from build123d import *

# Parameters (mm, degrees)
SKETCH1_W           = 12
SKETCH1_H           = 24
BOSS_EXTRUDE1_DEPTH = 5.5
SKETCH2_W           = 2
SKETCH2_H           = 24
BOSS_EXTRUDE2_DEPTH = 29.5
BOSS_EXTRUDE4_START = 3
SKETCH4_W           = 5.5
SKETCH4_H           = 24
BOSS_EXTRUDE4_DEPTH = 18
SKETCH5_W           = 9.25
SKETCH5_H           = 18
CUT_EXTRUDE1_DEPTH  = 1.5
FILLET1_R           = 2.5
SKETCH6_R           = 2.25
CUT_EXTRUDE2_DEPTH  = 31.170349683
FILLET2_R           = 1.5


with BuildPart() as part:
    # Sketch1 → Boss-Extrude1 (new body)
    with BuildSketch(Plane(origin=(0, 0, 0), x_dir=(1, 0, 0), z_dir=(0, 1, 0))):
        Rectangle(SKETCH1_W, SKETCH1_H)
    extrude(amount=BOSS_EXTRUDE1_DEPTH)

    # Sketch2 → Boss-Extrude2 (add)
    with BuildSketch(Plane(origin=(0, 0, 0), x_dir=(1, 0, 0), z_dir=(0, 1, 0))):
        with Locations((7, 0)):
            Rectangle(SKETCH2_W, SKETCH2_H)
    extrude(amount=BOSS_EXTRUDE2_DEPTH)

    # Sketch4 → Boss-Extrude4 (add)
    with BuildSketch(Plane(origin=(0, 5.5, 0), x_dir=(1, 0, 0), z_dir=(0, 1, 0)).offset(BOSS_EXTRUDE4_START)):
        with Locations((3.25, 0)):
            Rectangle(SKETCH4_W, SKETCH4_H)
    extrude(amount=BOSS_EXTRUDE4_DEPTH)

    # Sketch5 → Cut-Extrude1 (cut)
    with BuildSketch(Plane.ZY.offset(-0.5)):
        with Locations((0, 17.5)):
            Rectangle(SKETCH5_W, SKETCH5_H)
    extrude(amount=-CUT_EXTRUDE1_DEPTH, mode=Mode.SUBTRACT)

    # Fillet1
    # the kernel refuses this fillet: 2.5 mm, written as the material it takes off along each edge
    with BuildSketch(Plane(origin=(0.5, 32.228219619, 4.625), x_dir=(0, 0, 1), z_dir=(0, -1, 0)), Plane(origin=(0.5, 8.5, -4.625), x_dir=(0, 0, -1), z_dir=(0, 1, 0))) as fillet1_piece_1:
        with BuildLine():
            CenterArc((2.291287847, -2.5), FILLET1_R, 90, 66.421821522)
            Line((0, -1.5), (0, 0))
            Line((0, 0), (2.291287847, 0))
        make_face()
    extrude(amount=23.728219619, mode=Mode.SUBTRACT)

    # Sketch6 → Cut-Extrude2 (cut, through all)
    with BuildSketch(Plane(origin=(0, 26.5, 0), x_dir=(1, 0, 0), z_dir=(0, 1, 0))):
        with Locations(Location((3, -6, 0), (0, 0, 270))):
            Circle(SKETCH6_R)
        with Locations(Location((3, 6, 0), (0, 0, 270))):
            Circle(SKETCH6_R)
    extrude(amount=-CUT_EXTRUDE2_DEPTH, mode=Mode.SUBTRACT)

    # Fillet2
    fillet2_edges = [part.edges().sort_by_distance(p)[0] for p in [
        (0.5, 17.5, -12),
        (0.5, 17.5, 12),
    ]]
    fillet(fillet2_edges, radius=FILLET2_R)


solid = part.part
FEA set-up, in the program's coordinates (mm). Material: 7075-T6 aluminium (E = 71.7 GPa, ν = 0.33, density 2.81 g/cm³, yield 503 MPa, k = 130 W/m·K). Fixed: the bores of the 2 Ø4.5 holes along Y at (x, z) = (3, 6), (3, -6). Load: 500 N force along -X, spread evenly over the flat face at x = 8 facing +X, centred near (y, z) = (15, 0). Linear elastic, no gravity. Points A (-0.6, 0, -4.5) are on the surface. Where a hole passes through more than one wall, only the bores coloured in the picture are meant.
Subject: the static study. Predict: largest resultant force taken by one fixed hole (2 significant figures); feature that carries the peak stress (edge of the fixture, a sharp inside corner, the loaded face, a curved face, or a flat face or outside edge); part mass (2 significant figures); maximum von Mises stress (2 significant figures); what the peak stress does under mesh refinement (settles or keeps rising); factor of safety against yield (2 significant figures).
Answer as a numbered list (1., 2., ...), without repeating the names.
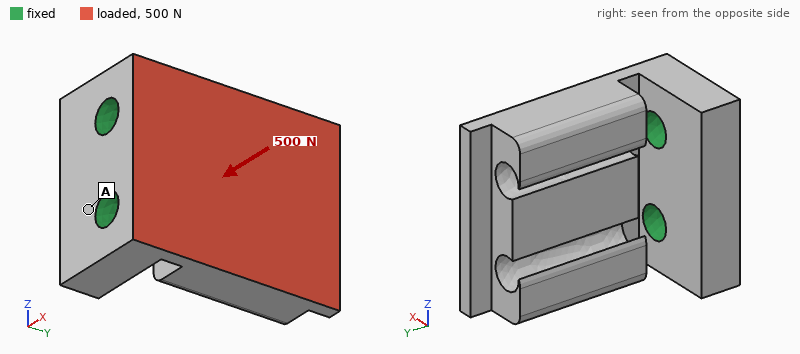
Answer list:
1. 250 N
2. the loaded face
3. 12 g
4. 260 MPa
5. settles
6. 1.9
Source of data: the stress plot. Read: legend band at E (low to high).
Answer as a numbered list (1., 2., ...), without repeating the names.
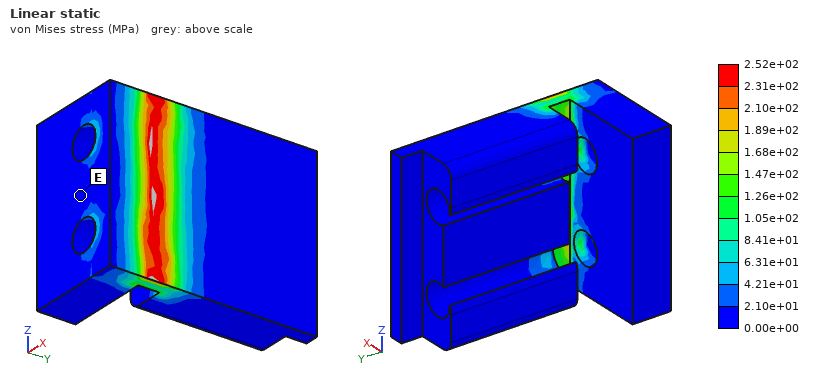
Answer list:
1. 0.00e+00 to 2.10e+01 MPa
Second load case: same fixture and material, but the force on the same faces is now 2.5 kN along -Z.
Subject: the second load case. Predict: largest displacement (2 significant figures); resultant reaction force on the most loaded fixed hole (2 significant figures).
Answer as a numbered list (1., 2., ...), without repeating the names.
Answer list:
1. 89 µm
2. 2.2 kN
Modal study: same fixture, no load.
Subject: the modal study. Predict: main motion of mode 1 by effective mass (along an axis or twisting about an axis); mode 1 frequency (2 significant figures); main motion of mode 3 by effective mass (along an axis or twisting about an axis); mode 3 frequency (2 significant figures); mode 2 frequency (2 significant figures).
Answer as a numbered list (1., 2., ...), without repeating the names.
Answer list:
1. along X
2. 2300 Hz
3. along Z
4. 12 kHz
5. 8600 Hz
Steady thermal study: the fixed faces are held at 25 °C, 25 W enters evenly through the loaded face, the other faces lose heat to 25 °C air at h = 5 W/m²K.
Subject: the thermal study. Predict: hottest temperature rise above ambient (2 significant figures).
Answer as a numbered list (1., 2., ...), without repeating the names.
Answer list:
1. 31 K
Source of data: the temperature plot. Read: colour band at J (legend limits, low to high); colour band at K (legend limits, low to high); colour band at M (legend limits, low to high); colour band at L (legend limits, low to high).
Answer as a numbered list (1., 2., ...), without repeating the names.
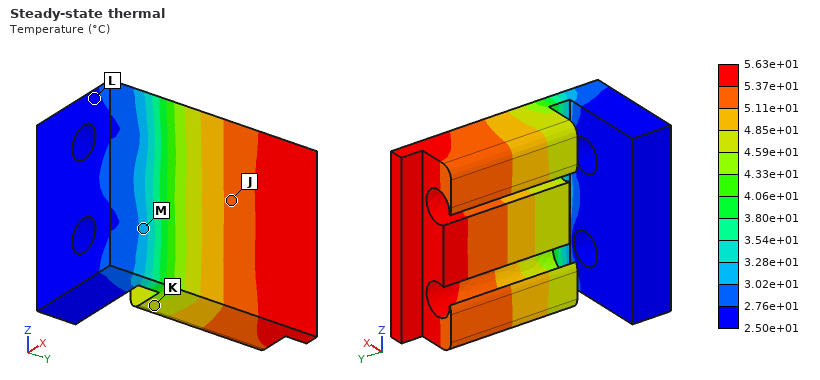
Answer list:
1. 5.11e+01 to 5.37e+01 °C
2. 4.59e+01 to 4.85e+01 °C
3. 3.02e+01 to 3.28e+01 °C
4. 2.50e+01 to 2.76e+01 °C
